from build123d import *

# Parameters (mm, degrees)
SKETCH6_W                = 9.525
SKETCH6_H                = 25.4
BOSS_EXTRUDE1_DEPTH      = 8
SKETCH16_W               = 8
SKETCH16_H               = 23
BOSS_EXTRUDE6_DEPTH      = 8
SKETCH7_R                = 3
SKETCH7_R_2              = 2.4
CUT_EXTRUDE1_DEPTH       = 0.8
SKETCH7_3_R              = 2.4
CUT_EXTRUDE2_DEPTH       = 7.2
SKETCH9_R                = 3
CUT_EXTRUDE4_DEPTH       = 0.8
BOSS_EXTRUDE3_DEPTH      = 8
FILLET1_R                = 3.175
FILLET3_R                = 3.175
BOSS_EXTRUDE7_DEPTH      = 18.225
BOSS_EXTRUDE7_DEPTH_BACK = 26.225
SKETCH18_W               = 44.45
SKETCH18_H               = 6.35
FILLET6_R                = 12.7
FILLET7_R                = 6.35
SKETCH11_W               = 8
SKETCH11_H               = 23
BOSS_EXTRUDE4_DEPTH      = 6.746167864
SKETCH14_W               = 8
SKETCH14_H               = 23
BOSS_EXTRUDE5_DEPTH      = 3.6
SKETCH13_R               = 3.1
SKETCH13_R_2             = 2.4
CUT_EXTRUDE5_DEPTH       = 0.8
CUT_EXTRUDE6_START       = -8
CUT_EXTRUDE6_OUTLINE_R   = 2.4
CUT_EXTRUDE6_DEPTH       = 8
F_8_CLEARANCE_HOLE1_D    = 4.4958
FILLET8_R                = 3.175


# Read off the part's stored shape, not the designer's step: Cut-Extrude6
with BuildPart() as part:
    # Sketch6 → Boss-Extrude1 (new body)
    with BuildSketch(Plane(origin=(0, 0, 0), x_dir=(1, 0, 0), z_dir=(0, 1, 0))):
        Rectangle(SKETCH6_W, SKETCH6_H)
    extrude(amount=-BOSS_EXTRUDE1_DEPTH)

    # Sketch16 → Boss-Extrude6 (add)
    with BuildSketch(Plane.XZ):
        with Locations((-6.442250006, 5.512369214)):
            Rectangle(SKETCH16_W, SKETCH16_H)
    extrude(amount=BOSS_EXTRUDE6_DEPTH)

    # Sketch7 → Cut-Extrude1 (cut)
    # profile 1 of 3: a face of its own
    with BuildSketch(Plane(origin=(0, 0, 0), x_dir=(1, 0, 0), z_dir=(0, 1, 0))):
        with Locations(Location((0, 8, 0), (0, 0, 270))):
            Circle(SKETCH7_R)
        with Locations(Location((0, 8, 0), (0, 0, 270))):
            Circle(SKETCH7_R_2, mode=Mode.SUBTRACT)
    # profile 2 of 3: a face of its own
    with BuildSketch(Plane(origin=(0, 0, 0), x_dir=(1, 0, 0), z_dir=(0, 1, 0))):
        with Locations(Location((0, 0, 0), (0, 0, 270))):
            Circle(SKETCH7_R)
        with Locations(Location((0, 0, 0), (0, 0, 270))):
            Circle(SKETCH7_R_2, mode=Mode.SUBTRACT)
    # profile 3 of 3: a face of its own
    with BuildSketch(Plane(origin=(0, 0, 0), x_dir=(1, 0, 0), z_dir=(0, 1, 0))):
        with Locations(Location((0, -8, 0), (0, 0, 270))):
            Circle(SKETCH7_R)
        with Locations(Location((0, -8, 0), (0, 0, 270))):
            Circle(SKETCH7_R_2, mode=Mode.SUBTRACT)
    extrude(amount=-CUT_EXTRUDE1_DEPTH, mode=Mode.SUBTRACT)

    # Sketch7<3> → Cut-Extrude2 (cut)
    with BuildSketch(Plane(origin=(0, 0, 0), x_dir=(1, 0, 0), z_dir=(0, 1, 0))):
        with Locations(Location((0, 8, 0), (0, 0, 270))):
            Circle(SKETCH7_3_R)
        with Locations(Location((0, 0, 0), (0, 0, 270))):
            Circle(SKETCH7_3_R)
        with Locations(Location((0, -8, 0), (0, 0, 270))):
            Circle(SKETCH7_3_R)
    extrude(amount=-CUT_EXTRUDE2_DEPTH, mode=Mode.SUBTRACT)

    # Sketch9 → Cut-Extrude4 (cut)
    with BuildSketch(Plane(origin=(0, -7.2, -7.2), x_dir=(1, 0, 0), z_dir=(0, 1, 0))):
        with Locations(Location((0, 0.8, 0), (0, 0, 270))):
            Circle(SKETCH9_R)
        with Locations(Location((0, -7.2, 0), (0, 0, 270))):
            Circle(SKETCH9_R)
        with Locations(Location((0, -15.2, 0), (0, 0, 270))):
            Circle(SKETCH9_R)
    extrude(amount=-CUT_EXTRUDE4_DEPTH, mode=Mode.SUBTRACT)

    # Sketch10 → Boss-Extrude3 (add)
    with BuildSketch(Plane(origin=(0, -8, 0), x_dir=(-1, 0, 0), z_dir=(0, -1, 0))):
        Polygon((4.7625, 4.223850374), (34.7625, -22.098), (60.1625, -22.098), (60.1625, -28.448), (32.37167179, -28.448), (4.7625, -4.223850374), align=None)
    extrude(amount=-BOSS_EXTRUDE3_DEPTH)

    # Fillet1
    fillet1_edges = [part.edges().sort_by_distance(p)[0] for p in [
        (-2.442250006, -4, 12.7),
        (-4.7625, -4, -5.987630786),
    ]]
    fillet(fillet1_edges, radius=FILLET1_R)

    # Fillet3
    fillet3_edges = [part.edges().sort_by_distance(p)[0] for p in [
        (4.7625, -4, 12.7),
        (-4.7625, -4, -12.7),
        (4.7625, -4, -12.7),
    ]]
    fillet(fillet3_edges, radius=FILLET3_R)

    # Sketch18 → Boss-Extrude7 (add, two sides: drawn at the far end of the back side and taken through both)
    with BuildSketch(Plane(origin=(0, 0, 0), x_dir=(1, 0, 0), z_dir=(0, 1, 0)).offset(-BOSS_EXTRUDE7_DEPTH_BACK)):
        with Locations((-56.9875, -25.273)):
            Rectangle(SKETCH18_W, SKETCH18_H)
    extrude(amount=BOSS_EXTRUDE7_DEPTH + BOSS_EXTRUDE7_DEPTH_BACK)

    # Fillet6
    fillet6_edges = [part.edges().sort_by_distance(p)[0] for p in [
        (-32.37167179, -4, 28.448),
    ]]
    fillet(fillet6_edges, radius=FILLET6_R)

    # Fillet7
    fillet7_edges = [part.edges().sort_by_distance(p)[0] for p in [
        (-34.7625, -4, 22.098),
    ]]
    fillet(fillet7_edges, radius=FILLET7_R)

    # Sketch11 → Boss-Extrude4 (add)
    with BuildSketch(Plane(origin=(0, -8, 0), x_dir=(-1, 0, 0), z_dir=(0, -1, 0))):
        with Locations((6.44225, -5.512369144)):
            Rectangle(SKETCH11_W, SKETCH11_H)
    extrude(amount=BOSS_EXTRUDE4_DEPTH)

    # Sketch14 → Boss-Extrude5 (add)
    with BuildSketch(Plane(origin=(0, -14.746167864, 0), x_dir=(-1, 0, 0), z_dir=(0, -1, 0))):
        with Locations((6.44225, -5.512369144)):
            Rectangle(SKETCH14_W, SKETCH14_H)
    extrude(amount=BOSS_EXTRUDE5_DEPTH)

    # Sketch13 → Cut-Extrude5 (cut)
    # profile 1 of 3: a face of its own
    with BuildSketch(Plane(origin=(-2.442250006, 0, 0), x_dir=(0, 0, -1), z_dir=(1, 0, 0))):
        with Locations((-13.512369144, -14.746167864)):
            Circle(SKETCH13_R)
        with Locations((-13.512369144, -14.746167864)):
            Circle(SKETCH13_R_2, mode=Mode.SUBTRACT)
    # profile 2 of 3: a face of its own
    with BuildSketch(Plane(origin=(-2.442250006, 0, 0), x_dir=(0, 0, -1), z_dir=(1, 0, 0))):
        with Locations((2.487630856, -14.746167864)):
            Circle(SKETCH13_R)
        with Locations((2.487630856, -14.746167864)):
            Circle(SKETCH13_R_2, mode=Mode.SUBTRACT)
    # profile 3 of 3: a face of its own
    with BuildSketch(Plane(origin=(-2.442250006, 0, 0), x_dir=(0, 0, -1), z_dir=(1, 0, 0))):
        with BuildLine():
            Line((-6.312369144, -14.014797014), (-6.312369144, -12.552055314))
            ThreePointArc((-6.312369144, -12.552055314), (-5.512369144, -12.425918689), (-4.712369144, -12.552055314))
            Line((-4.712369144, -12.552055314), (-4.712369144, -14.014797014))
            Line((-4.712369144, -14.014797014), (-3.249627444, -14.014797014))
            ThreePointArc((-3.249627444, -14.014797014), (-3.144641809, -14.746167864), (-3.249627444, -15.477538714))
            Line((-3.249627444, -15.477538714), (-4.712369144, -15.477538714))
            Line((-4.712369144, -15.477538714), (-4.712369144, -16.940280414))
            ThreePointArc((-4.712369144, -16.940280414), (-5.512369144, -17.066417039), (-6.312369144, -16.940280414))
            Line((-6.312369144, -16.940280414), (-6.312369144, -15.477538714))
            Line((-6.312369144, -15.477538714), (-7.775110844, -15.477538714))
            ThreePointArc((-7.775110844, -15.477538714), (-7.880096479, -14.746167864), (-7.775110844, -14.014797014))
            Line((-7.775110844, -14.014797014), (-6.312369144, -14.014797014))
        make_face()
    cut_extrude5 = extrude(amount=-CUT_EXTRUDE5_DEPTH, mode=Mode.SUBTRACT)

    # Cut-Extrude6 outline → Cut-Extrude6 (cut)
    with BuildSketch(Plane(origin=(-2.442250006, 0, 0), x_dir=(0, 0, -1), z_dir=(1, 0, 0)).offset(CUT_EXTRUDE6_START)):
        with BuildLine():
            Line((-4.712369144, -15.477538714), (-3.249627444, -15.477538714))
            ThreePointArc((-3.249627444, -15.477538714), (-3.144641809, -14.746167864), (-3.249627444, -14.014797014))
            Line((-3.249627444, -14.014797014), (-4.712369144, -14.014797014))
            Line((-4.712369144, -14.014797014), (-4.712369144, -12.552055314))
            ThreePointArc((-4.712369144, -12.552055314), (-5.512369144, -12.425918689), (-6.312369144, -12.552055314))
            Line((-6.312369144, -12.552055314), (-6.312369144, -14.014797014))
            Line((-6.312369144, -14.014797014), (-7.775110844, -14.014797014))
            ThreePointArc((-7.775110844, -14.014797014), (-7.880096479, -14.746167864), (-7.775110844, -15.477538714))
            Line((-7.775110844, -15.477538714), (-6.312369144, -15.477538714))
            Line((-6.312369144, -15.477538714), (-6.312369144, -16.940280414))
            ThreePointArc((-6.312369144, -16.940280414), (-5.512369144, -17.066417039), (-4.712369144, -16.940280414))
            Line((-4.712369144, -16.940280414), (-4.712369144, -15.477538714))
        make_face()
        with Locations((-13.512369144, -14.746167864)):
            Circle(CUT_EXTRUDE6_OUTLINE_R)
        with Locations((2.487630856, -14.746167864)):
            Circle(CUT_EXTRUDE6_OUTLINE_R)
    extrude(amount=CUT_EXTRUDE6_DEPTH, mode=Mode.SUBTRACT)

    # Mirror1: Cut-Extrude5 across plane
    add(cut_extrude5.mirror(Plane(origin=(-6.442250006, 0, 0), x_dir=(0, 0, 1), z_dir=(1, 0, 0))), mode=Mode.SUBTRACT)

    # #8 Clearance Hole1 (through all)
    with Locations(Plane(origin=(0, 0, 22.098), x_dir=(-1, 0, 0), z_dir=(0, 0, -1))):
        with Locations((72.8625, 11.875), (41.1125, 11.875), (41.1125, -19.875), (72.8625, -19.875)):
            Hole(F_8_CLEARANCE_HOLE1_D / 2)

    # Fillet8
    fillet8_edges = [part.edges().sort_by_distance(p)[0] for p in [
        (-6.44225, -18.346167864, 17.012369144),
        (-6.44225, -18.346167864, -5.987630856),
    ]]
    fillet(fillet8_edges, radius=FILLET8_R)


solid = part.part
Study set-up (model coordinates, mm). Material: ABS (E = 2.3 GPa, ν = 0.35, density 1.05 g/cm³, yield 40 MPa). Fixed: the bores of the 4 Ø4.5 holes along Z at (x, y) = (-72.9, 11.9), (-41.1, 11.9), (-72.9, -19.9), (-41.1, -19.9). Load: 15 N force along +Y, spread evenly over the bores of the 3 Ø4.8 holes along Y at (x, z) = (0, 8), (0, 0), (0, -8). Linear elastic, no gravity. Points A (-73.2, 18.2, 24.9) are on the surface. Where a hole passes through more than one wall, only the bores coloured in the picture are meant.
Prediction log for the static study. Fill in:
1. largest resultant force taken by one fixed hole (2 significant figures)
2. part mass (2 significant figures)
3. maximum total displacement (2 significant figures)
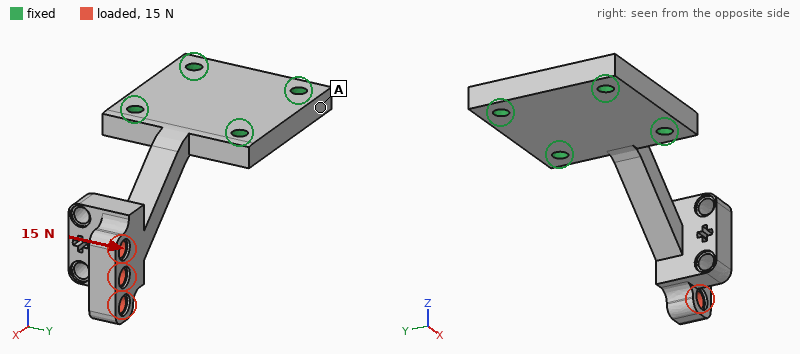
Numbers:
26 N
19 g
1.0 mm
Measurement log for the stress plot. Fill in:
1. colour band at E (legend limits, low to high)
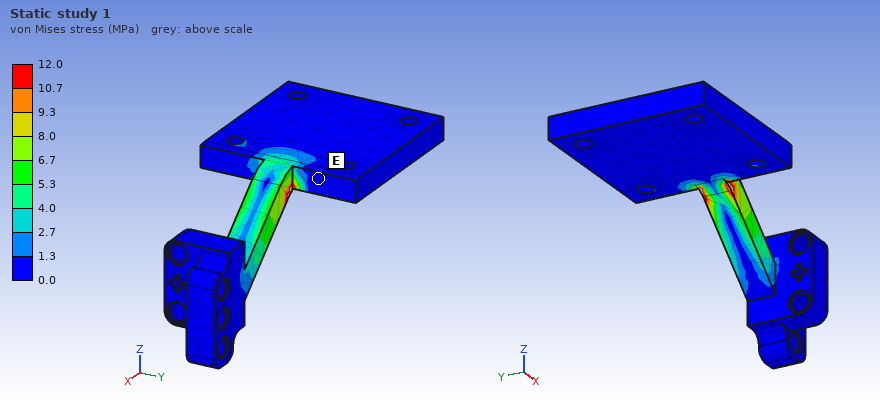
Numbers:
0.0 to 1.3 MPa
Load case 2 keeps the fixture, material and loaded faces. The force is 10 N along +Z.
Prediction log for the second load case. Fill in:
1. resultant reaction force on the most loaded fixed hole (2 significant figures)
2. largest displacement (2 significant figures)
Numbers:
8.9 N
1.1 mm
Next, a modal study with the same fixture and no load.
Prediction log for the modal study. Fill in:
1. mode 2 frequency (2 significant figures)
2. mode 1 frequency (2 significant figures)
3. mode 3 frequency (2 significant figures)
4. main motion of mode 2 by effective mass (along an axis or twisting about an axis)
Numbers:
380 Hz
270 Hz
950 Hz
along Y
